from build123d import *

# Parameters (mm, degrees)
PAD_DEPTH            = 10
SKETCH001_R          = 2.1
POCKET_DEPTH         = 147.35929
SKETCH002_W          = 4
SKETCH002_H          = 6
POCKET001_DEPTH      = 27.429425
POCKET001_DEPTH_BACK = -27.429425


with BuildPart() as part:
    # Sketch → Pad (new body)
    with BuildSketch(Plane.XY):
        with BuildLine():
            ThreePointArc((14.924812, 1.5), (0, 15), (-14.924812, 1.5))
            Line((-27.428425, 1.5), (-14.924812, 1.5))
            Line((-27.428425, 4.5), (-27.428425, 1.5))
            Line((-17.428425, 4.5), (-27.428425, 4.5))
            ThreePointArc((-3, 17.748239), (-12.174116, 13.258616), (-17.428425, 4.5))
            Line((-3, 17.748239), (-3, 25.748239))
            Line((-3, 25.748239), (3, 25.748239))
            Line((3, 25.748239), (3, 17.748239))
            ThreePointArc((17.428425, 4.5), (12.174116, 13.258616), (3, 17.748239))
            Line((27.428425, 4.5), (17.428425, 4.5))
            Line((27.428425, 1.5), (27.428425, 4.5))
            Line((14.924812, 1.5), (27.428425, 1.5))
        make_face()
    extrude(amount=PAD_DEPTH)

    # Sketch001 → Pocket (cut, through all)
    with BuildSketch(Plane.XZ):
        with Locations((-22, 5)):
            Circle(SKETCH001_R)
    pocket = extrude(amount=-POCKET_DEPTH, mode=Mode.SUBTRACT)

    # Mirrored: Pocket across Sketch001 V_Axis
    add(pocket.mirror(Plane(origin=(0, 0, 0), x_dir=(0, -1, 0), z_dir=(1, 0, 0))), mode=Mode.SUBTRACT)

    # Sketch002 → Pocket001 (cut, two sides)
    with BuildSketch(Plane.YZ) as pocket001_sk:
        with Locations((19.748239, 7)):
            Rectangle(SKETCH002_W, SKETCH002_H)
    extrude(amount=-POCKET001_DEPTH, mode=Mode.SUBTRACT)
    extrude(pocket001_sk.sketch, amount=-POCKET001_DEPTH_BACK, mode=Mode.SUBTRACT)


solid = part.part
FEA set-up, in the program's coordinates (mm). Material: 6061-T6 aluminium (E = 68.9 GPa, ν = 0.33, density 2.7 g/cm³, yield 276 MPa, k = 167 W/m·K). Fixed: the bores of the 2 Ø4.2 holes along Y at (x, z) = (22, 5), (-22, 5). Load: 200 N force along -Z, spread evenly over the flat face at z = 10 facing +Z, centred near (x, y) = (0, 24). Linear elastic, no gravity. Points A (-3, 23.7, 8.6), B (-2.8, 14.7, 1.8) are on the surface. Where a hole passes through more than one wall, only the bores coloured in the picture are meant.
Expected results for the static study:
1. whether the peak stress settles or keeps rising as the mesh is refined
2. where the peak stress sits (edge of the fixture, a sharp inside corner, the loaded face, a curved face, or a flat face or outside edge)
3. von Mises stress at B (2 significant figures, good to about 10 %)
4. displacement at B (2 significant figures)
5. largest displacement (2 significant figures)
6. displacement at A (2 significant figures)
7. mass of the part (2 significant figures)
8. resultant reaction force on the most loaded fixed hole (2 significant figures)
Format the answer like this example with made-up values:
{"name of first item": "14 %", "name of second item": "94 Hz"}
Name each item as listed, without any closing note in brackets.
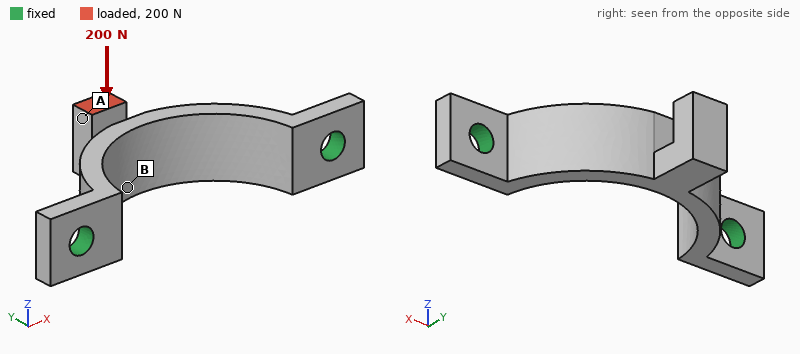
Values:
{"whether the peak stress settles or keeps rising as the mesh is refined": "keeps rising", "where the peak stress sits": "edge of the fixture", "von Mises stress at B": "46 MPa", "displacement at B": "0.057 mm", "largest displacement": "0.16 mm", "displacement at A": "0.14 mm", "mass of the part": "6.2 g", "resultant reaction force on the most loaded fixed hole": "100 N"}
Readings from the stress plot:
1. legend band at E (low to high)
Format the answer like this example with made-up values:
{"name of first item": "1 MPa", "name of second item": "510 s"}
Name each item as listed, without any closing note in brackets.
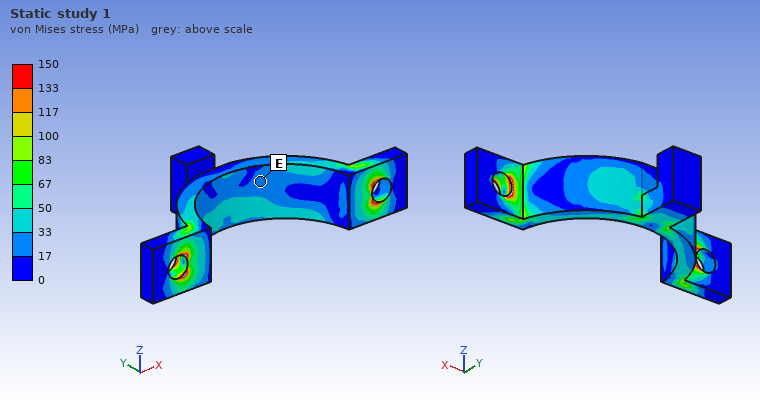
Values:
{"legend band at E": "17 to 33 MPa"}
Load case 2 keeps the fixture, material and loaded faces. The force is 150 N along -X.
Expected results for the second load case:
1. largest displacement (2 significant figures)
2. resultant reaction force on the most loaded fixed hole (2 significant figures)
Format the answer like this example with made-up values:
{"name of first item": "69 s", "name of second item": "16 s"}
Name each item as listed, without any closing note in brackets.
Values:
{"largest displacement": "57 µm", "resultant reaction force on the most loaded fixed hole": "110 N"}
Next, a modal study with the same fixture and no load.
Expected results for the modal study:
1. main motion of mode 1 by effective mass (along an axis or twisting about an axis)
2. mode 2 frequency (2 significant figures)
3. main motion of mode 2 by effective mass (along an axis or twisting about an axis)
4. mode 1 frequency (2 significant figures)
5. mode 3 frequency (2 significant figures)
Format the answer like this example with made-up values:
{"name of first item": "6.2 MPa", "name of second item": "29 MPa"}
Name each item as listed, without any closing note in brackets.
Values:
{"main motion of mode 1 by effective mass": "along Z", "mode 2 frequency": "12 kHz", "main motion of mode 2 by effective mass": "along X", "mode 1 frequency": "5400 Hz", "mode 3 frequency": "15 kHz"}
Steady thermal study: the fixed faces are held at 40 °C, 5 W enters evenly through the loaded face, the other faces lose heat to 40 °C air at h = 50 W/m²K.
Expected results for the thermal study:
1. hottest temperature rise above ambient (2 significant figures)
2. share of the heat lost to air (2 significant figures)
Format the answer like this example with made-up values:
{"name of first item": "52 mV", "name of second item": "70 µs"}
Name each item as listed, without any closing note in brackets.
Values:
{"hottest temperature rise above ambient": "27 K", "share of the heat lost to air": "13 %"}
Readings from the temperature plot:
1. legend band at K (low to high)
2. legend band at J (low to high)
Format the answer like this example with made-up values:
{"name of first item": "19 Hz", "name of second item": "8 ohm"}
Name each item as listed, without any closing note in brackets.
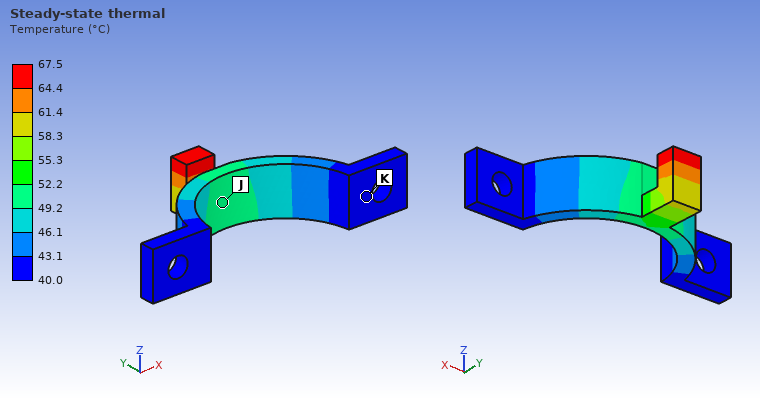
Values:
{"legend band at K": "40.0 to 43.1 °C", "legend band at J": "49.2 to 52.2 °C"}
